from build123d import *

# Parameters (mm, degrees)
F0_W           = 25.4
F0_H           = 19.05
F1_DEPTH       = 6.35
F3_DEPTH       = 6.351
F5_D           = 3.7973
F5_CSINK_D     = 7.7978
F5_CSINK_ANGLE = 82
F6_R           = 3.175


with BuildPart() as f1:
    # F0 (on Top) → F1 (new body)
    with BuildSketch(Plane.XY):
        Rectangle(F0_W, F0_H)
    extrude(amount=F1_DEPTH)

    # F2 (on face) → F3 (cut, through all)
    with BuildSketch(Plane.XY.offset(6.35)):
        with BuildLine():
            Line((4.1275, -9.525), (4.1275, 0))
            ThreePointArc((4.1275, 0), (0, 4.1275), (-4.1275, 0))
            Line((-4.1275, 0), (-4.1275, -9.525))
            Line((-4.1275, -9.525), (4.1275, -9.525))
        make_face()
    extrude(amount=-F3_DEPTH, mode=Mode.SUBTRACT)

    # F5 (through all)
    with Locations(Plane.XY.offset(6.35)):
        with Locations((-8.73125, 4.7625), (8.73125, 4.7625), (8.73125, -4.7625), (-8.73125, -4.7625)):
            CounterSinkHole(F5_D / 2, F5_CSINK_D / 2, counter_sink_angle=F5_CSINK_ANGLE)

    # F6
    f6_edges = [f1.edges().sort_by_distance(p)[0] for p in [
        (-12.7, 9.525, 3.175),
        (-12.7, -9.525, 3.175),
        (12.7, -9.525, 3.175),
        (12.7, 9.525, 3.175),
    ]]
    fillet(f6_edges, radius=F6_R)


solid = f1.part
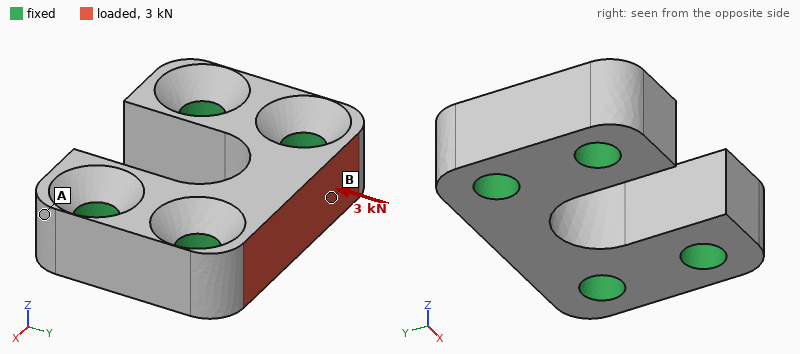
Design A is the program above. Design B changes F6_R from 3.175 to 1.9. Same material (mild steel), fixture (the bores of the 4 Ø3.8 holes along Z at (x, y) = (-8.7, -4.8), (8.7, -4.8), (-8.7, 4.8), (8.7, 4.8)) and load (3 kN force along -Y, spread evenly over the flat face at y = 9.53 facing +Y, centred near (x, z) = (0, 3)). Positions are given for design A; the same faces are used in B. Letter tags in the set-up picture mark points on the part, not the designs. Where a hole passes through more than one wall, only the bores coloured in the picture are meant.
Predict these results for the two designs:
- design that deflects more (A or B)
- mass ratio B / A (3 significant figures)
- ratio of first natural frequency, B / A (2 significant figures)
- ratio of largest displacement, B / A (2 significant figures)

A
1.02
1.00
0.89
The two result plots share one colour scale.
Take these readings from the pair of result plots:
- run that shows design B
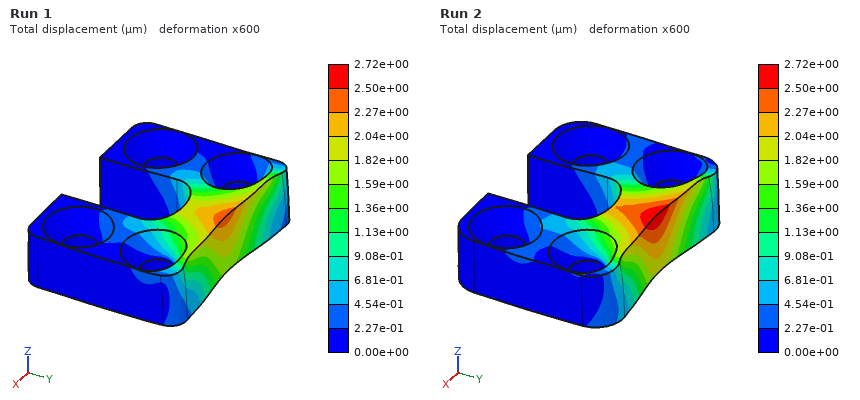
Run 1
